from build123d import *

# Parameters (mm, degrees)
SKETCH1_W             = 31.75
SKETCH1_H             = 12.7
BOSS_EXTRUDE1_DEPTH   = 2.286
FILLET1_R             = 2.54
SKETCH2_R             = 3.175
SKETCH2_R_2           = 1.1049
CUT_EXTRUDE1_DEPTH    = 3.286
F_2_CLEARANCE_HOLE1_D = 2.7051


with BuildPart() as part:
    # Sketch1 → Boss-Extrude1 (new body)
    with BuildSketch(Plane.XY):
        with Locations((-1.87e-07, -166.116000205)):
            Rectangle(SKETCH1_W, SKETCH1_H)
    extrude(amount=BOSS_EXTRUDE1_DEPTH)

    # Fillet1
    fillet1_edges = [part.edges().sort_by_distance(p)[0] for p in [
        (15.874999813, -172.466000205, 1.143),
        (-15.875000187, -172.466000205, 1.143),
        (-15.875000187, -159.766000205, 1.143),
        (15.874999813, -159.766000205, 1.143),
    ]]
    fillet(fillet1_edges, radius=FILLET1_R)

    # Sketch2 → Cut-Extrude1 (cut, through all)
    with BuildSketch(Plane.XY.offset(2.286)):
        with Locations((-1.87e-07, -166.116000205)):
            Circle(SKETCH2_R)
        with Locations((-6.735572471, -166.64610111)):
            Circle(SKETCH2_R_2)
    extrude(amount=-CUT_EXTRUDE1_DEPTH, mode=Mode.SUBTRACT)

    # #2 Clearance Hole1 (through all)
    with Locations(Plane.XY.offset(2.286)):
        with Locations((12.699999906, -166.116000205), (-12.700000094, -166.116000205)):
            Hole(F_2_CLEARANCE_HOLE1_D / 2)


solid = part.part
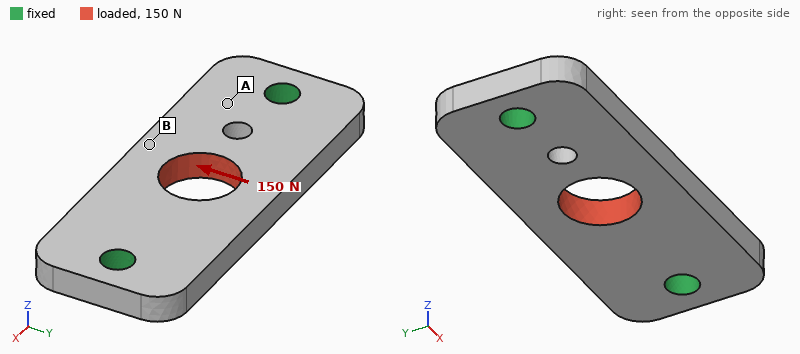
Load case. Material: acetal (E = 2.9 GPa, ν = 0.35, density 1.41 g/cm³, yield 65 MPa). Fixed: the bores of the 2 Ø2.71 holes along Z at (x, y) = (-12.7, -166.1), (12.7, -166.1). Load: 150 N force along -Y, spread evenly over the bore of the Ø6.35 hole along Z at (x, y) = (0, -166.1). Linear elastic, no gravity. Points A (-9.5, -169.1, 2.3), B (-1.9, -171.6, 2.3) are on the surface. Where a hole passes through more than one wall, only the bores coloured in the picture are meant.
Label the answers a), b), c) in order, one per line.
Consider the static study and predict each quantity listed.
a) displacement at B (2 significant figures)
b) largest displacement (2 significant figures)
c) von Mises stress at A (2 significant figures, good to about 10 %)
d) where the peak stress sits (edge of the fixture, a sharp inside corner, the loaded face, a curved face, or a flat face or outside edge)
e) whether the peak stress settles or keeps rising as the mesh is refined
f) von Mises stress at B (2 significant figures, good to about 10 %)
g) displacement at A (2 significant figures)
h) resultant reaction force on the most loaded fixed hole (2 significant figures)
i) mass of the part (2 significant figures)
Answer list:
a) 58 µm
b) 64 µm
c) 4.4 MPa
d) edge of the fixture
e) keeps rising
f) 9.4 MPa
g) 17 µm
h) 76 N
i) 1.1 g
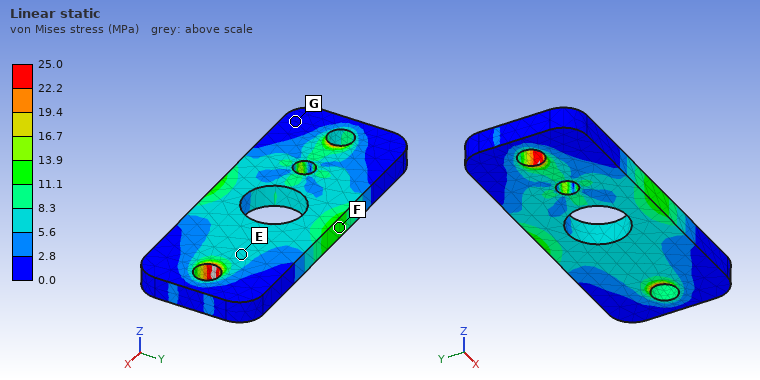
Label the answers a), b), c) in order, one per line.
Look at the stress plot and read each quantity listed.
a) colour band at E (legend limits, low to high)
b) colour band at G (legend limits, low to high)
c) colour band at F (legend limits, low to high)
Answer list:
a) 5.6 to 8.3 MPa
b) 0.0 to 2.8 MPa
c) 11.1 to 13.9 MPa
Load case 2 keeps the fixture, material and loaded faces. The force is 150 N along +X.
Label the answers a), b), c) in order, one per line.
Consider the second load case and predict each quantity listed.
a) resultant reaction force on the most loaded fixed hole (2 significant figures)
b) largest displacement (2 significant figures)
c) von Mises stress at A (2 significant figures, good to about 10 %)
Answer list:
a) 77 N
b) 17 µm
c) 3.6 MPa
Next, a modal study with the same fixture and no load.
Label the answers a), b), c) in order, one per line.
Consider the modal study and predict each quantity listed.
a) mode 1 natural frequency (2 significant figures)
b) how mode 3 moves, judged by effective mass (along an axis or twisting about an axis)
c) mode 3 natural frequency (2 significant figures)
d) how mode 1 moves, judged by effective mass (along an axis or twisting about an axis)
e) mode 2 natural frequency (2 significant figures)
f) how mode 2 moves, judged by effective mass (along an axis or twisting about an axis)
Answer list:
a) 5100 Hz
b) twisting about Y
c) 12 kHz
d) along Z
e) 6000 Hz
f) twisting about X
